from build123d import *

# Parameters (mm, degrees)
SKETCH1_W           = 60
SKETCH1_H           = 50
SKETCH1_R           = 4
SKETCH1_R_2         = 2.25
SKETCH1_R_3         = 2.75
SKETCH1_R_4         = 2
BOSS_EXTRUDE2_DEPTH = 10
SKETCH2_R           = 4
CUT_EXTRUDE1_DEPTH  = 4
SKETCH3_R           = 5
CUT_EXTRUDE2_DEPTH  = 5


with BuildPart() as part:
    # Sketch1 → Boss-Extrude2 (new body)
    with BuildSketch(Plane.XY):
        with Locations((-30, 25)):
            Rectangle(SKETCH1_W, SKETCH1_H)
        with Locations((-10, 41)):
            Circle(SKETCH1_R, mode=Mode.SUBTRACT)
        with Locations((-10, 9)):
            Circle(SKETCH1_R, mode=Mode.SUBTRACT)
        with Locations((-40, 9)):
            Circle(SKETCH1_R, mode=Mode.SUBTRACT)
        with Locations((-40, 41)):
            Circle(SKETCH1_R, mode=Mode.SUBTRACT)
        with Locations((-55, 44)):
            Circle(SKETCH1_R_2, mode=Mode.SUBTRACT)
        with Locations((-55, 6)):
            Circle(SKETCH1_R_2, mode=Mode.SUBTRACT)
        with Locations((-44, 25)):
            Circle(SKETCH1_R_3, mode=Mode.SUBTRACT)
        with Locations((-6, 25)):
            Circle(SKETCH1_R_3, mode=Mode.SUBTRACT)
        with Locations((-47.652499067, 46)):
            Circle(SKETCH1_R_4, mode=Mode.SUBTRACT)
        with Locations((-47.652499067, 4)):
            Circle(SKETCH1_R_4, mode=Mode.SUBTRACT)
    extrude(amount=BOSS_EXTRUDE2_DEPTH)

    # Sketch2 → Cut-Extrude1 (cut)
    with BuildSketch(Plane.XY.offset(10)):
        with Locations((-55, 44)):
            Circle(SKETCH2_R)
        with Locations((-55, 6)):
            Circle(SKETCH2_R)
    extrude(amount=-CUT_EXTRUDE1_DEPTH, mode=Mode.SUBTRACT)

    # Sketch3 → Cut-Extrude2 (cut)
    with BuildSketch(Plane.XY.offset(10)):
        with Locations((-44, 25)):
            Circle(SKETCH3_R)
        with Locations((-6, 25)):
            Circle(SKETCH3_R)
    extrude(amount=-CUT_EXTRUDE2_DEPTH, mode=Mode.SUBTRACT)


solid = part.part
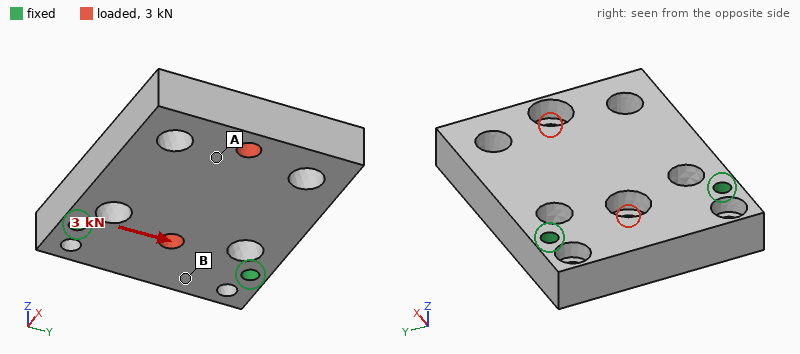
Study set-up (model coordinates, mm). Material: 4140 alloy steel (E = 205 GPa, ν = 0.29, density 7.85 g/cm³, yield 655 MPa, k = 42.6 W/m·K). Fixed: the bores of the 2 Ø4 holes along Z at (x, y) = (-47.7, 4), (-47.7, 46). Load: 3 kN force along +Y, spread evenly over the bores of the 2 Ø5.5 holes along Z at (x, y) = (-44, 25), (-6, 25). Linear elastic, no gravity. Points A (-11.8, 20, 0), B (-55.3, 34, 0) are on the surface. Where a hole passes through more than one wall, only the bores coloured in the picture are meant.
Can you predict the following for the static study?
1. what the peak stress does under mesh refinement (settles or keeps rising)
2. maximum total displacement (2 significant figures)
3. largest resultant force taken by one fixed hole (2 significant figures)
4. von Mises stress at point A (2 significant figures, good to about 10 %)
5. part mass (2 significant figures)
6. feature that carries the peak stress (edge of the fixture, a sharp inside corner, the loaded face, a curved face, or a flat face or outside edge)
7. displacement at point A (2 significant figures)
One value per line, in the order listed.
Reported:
keeps rising
7.9 µm
2.2 kN
16 MPa
210 g
edge of the fixture
5.5 µm
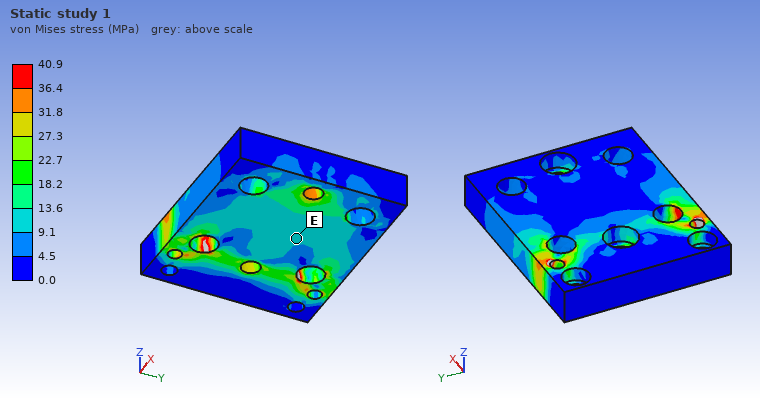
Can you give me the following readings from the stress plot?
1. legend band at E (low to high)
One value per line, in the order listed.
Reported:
9.1 to 13.6 MPa
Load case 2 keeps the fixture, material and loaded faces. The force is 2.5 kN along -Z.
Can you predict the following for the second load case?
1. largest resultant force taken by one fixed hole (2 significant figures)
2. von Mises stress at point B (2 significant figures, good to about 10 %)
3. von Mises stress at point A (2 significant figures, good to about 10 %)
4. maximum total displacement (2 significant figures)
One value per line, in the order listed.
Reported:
1.3 kN
24 MPa
33 MPa
94 µm
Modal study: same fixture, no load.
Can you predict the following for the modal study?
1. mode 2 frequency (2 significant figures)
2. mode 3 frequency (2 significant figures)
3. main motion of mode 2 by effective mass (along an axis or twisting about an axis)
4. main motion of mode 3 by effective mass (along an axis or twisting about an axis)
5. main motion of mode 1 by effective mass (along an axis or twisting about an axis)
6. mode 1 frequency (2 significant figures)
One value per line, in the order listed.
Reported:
7200 Hz
9800 Hz
twisting about X
along Y
along Z
2700 Hz
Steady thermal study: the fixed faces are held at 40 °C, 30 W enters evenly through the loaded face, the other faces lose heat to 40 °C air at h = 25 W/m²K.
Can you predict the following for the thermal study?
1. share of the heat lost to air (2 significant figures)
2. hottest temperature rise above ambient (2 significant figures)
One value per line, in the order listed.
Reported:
20 %
61 K
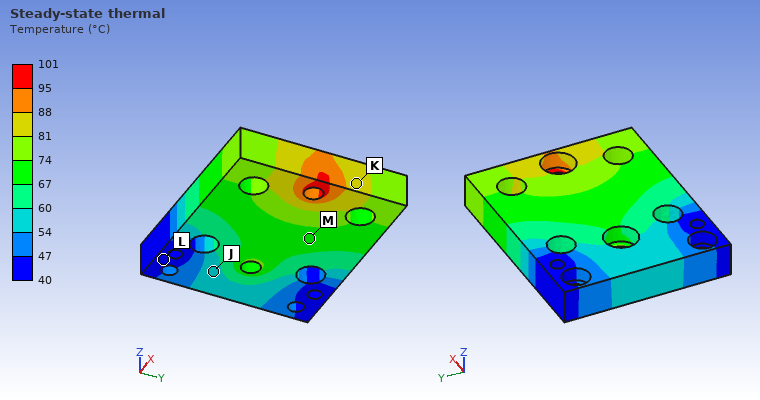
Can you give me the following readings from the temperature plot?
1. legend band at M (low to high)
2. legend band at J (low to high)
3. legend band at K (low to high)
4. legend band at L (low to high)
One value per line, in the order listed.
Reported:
67 to 74 °C
54 to 60 °C
81 to 88 °C
40 to 47 °C
